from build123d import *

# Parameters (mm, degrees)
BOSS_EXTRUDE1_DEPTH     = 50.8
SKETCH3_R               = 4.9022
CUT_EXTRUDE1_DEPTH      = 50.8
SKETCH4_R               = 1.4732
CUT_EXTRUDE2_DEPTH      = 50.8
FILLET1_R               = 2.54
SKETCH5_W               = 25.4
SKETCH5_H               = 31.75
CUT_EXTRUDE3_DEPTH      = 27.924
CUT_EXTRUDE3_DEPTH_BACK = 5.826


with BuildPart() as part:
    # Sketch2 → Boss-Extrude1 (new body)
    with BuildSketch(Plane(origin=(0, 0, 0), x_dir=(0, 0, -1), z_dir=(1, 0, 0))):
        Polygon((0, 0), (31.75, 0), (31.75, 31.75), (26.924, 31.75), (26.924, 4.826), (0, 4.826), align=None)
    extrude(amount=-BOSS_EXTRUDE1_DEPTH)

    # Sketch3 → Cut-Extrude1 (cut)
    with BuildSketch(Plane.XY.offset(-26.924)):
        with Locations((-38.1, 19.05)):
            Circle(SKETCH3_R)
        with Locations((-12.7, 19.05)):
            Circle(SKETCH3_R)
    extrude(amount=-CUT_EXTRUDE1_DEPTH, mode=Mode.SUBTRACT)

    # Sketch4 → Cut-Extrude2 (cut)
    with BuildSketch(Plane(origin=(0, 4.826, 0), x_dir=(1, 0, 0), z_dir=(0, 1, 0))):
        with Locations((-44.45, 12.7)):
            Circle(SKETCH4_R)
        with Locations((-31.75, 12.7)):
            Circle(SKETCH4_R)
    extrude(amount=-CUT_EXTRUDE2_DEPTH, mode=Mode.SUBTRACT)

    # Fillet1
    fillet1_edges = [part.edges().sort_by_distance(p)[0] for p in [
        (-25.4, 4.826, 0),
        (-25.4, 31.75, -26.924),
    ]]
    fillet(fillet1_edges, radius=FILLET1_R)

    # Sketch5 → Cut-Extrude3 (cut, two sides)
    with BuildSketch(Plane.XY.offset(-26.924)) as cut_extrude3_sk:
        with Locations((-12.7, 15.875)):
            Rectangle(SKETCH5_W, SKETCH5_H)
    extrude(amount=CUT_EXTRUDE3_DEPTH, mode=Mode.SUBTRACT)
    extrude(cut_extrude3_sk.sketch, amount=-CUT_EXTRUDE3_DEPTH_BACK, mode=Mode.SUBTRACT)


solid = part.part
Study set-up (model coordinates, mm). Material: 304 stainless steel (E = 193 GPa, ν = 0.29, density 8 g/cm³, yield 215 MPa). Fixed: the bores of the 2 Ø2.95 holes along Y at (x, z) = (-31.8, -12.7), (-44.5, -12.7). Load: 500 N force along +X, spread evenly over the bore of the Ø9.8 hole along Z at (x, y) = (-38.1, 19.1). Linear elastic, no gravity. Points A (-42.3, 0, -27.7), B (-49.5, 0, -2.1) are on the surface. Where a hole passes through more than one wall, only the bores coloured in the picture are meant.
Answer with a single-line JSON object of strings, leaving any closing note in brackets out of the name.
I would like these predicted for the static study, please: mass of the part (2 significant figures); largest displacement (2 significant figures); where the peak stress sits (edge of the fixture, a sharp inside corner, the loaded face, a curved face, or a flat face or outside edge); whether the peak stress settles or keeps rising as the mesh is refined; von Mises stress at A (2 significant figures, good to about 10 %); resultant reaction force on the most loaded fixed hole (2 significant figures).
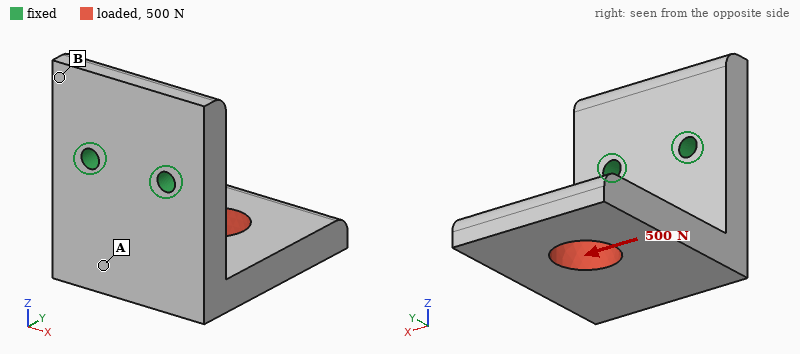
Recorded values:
{"mass of the part": "54 g", "largest displacement": "42 µm", "where the peak stress sits": "edge of the fixture", "whether the peak stress settles or keeps rising as the mesh is refined": "keeps rising", "von Mises stress at A": "34 MPa", "resultant reaction force on the most loaded fixed hole": "780 N"}
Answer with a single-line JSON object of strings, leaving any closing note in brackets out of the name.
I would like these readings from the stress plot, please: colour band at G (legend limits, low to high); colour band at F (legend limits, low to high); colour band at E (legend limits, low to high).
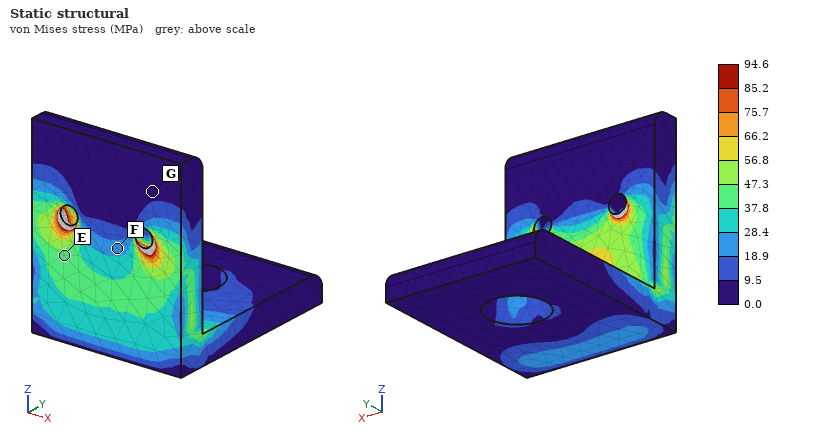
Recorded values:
{"colour band at G": "0.0 to 9.5 MPa", "colour band at F": "18.9 to 28.4 MPa", "colour band at E": "37.8 to 47.3 MPa"}
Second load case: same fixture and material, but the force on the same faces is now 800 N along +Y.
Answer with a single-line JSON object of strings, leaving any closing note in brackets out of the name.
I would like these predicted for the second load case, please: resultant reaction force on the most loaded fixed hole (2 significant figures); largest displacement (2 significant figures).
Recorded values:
{"resultant reaction force on the most loaded fixed hole": "400 N", "largest displacement": "80 µm"}
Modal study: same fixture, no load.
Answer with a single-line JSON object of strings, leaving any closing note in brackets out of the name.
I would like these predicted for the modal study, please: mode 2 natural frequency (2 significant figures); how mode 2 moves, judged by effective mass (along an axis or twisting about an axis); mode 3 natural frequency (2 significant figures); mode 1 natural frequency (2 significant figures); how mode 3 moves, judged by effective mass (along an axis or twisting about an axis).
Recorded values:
{"mode 2 natural frequency": "4200 Hz", "how mode 2 moves, judged by effective mass": "along X", "mode 3 natural frequency": "7300 Hz", "mode 1 natural frequency": "2500 Hz", "how mode 3 moves, judged by effective mass": "along Y"}
